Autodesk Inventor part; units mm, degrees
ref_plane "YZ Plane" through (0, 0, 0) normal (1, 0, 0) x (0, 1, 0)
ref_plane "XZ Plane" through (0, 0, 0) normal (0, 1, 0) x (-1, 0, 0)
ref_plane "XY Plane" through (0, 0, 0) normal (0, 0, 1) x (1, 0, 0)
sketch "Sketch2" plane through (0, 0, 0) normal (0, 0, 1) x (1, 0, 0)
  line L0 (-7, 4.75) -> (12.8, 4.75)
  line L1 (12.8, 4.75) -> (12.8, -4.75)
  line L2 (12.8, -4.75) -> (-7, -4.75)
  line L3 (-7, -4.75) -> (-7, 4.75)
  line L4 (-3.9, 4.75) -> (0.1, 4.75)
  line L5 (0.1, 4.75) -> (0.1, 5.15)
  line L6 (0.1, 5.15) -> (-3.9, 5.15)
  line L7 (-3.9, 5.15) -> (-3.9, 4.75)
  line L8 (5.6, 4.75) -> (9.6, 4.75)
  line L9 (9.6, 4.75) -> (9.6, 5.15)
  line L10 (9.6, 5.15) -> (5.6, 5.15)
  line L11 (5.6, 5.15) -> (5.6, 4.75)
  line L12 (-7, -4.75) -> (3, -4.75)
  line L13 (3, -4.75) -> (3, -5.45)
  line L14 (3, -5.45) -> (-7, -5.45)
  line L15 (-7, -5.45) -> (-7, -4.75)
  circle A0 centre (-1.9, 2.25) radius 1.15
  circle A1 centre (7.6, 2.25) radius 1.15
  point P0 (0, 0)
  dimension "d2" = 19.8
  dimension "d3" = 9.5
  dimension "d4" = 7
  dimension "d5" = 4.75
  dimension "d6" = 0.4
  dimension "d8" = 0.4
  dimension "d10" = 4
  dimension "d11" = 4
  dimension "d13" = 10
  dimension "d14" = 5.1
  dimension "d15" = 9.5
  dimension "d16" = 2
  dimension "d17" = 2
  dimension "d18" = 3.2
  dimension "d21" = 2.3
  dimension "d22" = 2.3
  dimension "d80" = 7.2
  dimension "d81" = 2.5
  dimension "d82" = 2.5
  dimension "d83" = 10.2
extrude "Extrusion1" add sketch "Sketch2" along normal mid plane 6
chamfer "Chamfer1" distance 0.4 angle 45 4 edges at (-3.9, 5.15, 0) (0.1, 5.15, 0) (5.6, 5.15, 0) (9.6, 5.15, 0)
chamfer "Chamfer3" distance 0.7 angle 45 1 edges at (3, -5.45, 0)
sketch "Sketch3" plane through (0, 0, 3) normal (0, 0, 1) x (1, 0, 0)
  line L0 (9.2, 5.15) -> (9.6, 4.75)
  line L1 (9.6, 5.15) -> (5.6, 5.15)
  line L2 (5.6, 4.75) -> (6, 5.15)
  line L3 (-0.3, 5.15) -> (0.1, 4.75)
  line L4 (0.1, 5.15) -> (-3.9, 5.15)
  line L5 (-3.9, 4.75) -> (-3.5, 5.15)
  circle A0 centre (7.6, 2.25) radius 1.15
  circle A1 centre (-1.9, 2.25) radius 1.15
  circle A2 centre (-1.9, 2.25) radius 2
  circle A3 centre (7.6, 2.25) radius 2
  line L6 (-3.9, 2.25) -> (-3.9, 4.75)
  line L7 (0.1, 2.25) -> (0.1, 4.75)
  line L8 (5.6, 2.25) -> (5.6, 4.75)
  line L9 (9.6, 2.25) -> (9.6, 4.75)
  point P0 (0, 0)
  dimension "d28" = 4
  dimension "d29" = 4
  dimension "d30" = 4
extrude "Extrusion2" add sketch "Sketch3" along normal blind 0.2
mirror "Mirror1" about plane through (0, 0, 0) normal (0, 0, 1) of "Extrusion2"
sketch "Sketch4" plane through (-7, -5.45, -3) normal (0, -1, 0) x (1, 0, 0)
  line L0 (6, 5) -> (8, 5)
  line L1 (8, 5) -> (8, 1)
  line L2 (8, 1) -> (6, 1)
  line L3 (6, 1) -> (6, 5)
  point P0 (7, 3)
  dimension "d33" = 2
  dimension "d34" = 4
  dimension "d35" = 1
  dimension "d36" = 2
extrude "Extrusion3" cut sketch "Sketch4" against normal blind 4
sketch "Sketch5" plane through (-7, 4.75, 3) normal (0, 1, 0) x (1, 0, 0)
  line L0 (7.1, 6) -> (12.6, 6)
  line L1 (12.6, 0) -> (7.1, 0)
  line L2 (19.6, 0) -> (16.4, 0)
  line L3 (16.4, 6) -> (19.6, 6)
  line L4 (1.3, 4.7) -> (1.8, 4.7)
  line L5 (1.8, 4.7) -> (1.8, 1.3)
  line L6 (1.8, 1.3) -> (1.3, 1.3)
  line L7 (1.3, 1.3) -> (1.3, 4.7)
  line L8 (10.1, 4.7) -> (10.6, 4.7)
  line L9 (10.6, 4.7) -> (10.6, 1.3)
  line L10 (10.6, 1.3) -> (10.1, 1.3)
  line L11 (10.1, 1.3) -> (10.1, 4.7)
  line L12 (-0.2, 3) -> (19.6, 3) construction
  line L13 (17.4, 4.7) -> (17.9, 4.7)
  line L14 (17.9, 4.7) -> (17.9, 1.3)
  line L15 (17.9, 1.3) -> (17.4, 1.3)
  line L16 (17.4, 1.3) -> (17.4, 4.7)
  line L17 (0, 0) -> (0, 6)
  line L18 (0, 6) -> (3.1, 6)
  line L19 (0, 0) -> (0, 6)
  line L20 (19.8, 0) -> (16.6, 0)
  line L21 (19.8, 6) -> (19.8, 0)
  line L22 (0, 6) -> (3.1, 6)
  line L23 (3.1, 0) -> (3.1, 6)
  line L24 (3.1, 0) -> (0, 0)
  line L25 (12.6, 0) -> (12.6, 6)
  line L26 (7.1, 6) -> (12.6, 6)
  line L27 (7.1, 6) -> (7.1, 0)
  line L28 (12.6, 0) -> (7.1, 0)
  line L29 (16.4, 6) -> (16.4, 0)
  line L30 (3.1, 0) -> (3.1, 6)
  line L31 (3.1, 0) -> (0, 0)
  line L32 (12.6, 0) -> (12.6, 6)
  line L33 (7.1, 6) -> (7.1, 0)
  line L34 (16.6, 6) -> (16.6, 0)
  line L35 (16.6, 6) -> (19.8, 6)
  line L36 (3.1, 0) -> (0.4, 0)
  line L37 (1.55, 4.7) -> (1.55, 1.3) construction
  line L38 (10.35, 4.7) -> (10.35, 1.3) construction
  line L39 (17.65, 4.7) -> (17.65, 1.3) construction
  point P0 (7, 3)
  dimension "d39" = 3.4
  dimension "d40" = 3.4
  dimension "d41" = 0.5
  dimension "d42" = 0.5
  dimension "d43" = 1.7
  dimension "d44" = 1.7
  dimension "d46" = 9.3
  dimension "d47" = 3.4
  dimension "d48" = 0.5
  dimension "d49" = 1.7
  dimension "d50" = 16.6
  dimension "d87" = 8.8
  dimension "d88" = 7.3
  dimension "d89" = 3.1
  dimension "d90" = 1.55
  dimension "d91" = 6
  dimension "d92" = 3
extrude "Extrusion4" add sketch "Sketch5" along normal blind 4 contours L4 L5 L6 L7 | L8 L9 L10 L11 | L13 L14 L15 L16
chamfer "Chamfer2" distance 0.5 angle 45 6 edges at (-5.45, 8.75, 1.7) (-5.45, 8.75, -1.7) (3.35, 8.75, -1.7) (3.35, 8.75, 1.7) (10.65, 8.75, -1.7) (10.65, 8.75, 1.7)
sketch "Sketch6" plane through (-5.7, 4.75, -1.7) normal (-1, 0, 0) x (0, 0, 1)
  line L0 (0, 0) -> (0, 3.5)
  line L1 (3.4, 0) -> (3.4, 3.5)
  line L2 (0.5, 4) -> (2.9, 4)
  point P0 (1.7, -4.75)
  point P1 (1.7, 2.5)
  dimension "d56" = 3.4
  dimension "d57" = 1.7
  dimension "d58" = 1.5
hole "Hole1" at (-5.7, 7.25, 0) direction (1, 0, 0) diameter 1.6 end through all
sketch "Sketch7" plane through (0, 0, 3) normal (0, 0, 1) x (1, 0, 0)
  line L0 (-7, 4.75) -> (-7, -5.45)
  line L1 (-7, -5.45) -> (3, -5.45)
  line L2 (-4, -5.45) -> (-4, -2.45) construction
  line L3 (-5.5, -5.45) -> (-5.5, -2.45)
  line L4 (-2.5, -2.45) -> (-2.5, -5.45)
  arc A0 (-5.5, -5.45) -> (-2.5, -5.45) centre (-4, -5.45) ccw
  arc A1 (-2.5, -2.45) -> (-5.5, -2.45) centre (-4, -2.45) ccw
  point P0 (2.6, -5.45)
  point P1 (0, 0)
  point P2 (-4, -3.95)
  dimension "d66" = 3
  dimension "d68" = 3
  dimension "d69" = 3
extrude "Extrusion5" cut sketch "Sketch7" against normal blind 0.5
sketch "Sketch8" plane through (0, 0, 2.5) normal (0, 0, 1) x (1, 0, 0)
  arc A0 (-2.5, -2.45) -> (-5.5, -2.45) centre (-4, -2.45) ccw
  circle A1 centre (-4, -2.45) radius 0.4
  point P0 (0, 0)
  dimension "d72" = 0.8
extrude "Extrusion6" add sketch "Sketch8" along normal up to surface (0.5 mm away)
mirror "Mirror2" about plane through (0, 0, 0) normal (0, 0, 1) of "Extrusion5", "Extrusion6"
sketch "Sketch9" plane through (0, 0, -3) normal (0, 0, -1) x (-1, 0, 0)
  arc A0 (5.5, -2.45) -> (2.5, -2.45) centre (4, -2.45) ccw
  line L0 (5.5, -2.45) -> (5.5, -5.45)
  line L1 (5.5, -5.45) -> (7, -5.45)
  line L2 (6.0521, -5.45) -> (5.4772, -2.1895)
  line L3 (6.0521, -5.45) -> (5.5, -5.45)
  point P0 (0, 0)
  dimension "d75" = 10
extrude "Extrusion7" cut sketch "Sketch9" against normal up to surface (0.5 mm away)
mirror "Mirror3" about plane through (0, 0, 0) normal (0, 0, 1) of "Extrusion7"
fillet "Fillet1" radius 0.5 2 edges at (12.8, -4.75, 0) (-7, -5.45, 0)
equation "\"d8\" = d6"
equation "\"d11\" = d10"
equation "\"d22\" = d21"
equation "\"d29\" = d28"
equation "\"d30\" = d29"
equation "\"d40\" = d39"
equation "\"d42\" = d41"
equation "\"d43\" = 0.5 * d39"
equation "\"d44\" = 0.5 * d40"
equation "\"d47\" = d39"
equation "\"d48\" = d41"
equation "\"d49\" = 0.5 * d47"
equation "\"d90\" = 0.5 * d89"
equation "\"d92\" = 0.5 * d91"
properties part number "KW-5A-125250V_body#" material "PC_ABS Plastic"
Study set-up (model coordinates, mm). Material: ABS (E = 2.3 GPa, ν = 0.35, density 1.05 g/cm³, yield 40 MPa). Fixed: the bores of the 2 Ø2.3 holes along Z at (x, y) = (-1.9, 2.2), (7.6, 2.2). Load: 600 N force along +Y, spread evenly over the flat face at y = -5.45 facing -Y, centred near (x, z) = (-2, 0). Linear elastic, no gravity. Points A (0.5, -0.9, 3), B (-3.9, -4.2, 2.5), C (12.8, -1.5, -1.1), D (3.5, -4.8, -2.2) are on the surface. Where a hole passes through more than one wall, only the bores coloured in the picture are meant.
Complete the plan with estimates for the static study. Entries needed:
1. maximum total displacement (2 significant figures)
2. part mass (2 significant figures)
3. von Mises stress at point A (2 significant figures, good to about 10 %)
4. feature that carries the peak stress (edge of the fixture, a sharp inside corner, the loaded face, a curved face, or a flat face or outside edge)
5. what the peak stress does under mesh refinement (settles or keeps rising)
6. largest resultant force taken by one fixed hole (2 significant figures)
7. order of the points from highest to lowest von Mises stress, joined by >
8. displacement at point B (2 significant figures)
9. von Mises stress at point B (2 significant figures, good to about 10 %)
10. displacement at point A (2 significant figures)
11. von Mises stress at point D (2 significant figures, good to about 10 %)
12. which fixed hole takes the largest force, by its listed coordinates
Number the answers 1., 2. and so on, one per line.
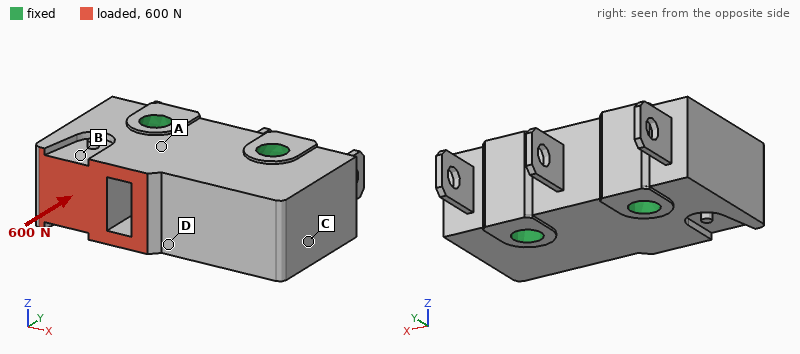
1. 79 µm
2. 1.2 g
3. 11 MPa
4. edge of the fixture
5. keeps rising
6. 580 N
7. B > A > D > C
8. 63 µm
9. 16 MPa
10. 14 µm
11. 5.7 MPa
12. (-1.9, 2.2)
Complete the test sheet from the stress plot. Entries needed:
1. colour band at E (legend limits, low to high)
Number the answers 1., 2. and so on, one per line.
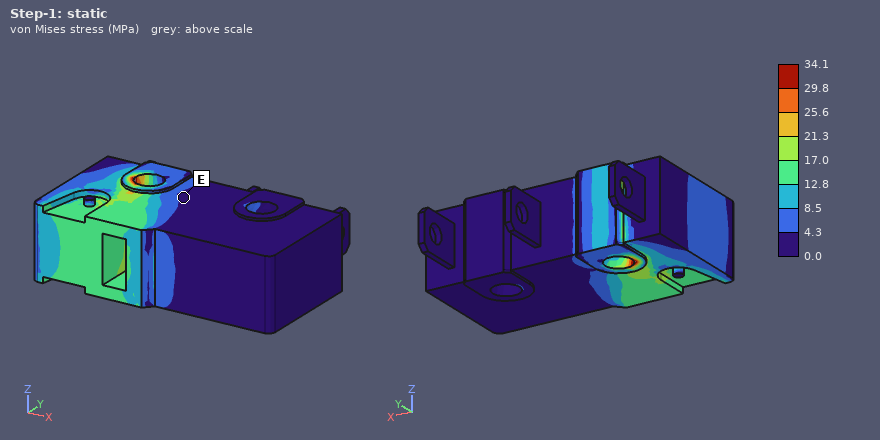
1. 0.0 to 4.3 MPa
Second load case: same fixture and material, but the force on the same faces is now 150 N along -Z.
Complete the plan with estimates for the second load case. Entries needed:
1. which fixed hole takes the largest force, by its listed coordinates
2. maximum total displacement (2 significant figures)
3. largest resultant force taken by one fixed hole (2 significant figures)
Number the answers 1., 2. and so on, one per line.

1. (-1.9, 2.2)
2. 0.10 mm
3. 130 N
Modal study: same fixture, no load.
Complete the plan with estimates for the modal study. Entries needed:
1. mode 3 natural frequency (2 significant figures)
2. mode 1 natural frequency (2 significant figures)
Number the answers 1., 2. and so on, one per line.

1. 7800 Hz
2. 7800 Hz
